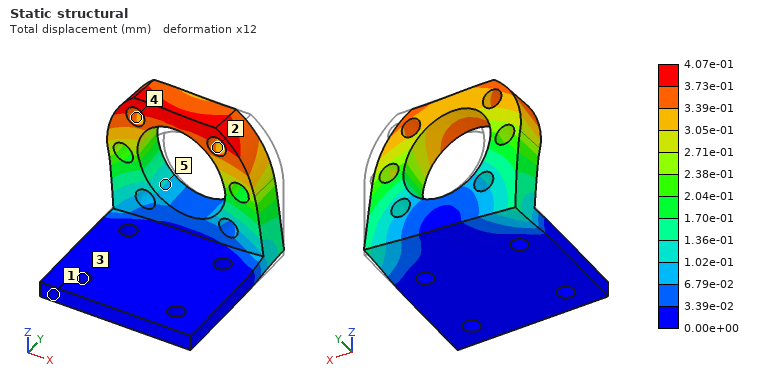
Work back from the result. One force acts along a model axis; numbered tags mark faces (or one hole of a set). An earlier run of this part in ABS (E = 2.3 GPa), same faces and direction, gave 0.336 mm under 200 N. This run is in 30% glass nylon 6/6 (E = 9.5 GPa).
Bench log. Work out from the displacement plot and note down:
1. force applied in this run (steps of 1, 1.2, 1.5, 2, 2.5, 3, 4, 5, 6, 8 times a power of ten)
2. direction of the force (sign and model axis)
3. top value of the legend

1 kN
-X
4.07e-01 mm
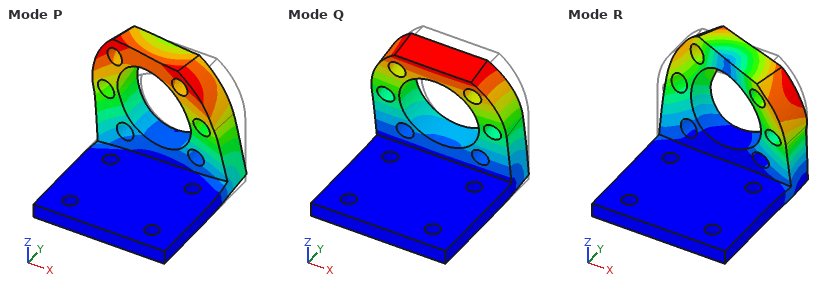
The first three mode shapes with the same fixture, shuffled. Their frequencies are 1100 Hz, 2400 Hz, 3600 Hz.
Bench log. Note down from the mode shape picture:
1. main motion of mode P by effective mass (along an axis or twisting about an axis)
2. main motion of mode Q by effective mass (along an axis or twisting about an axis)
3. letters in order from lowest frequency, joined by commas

along X
along Y
Q, P, R
